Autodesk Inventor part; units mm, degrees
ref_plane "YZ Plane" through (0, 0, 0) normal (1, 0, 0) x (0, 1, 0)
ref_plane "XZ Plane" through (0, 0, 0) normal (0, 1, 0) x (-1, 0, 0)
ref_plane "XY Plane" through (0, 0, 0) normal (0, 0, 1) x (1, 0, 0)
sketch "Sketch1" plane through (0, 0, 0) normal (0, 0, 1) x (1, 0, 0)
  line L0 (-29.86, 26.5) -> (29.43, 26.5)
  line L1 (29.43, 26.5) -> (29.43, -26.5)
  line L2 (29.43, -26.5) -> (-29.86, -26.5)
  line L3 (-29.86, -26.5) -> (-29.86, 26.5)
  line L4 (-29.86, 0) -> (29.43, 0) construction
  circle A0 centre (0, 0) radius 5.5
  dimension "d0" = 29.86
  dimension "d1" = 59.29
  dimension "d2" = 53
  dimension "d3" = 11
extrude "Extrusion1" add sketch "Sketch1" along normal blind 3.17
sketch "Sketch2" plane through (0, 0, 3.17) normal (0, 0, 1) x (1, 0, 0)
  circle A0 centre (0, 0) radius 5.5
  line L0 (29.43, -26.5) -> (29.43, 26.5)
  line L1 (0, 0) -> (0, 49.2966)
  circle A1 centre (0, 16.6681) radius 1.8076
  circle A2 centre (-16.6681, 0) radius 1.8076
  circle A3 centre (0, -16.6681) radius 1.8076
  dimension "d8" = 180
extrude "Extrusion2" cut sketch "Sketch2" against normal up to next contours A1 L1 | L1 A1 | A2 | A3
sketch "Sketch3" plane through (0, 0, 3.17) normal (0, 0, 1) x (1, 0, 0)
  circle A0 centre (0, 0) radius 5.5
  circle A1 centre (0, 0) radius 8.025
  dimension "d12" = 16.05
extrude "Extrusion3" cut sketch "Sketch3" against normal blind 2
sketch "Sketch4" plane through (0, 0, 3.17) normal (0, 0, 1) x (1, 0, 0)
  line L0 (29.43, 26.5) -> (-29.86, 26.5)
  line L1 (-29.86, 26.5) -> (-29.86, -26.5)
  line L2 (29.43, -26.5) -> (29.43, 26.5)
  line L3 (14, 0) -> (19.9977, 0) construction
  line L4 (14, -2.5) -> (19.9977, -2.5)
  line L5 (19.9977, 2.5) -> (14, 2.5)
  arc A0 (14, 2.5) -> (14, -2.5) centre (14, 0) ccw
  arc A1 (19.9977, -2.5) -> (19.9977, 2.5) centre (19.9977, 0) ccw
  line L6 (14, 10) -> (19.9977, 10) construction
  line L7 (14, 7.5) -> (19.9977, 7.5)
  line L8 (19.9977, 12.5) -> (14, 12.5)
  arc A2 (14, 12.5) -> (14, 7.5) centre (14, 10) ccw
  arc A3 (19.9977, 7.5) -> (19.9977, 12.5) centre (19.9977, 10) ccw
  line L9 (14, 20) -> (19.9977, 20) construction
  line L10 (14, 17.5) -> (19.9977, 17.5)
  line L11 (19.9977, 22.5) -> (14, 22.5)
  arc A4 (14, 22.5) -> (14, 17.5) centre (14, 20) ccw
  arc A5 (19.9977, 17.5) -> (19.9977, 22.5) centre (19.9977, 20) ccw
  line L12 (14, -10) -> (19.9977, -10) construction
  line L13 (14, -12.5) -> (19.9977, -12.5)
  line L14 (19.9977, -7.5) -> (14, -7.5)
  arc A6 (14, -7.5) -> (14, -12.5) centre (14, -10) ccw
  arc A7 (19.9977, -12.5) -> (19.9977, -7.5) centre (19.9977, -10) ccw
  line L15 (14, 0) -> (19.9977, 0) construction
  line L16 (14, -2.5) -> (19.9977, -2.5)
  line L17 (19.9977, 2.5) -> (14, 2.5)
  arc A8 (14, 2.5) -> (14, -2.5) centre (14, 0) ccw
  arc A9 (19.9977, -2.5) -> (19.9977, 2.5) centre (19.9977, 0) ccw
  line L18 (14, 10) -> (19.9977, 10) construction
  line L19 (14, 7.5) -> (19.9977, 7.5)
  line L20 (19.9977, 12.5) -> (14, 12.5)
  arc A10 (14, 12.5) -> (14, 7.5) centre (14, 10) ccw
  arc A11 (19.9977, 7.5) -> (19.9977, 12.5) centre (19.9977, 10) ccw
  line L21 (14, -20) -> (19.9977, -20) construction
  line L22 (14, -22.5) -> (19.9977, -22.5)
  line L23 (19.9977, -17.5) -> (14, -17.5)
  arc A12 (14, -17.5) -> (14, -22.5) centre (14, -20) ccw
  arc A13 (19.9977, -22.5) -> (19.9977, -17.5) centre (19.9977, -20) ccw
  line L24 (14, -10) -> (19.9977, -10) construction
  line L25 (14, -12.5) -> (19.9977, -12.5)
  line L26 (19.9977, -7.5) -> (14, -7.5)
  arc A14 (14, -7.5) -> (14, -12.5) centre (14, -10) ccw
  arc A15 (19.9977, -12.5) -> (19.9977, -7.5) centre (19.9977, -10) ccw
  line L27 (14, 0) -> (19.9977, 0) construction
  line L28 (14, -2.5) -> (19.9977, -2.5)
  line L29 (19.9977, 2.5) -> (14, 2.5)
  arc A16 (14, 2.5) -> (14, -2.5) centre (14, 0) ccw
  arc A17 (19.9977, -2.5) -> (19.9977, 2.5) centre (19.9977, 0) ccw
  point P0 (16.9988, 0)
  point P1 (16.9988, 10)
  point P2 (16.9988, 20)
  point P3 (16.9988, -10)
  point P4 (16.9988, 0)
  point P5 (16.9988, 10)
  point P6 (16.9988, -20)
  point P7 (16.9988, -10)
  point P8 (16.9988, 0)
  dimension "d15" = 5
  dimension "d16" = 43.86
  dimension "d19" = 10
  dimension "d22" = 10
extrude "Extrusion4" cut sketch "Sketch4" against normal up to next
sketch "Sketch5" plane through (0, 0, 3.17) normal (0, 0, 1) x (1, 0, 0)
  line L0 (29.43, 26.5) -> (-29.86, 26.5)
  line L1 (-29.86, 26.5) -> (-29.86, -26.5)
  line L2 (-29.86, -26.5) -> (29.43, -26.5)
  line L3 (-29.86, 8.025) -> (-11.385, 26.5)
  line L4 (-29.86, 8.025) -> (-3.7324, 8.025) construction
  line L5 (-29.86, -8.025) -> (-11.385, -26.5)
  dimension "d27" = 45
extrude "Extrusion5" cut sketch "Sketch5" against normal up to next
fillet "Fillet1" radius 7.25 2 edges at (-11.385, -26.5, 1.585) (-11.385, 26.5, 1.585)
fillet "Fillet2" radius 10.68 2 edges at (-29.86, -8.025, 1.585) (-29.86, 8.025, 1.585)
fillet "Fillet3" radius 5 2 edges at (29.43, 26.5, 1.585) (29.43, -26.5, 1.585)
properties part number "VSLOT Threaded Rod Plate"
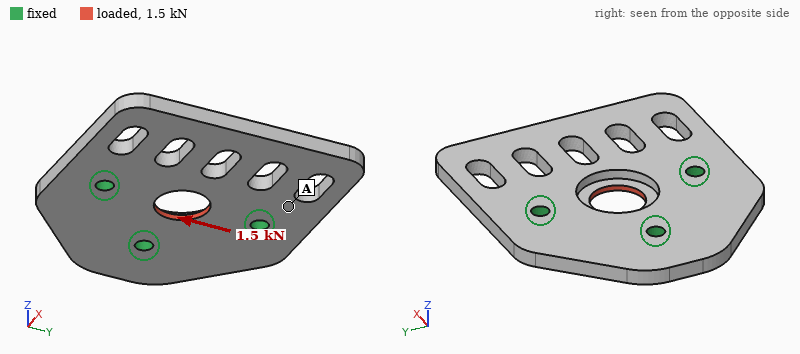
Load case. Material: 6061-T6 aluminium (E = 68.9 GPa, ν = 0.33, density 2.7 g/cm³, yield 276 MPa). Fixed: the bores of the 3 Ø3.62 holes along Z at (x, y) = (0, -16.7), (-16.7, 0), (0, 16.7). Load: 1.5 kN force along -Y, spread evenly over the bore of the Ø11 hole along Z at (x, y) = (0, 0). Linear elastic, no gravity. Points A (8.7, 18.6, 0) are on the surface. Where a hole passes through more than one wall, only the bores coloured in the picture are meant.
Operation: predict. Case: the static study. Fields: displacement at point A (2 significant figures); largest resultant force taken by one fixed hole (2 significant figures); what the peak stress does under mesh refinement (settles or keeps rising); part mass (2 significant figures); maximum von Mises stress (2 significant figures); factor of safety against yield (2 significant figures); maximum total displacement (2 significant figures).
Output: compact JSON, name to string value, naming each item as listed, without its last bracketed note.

{"displacement at point A": "2.1 µm", "largest resultant force taken by one fixed hole": "640 N", "what the peak stress does under mesh refinement": "settles", "part mass": "20 g", "maximum von Mises stress": "68 MPa", "factor of safety against yield": "4.1", "maximum total displacement": "7.0 µm"}
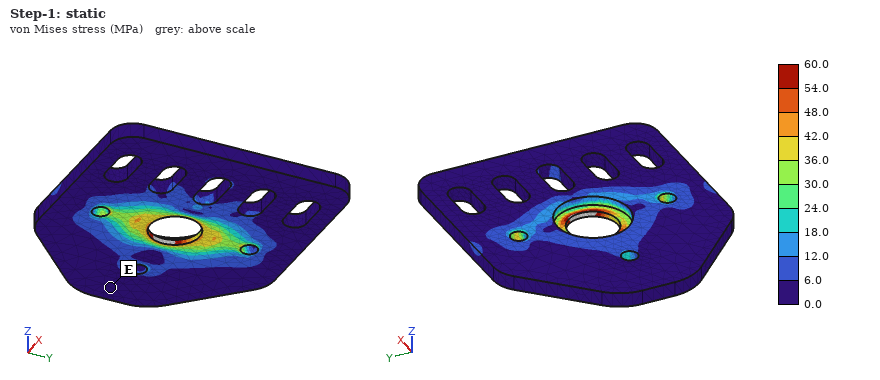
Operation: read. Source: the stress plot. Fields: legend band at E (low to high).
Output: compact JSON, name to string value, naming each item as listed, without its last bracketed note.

{"legend band at E": "0.0 to 6.0 MPa"}
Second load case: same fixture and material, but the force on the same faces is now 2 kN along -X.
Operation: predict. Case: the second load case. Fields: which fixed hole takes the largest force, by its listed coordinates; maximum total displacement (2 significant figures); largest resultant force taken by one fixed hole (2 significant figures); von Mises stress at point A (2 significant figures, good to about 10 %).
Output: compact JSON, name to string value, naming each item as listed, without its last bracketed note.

{"which fixed hole takes the largest force, by its listed coordinates": "(-16.7, 0)", "maximum total displacement": "30 µm", "largest resultant force taken by one fixed hole": "750 N", "von Mises stress at point A": "12 MPa"}
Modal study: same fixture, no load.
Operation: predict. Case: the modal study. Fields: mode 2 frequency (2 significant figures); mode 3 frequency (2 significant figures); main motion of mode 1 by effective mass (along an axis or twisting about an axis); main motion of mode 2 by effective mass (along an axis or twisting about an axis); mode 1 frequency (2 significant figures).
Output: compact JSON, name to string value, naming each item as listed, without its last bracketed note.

{"mode 2 frequency": "4600 Hz", "mode 3 frequency": "8100 Hz", "main motion of mode 1 by effective mass": "along Z", "main motion of mode 2 by effective mass": "twisting about X", "mode 1 frequency": "2700 Hz"}
